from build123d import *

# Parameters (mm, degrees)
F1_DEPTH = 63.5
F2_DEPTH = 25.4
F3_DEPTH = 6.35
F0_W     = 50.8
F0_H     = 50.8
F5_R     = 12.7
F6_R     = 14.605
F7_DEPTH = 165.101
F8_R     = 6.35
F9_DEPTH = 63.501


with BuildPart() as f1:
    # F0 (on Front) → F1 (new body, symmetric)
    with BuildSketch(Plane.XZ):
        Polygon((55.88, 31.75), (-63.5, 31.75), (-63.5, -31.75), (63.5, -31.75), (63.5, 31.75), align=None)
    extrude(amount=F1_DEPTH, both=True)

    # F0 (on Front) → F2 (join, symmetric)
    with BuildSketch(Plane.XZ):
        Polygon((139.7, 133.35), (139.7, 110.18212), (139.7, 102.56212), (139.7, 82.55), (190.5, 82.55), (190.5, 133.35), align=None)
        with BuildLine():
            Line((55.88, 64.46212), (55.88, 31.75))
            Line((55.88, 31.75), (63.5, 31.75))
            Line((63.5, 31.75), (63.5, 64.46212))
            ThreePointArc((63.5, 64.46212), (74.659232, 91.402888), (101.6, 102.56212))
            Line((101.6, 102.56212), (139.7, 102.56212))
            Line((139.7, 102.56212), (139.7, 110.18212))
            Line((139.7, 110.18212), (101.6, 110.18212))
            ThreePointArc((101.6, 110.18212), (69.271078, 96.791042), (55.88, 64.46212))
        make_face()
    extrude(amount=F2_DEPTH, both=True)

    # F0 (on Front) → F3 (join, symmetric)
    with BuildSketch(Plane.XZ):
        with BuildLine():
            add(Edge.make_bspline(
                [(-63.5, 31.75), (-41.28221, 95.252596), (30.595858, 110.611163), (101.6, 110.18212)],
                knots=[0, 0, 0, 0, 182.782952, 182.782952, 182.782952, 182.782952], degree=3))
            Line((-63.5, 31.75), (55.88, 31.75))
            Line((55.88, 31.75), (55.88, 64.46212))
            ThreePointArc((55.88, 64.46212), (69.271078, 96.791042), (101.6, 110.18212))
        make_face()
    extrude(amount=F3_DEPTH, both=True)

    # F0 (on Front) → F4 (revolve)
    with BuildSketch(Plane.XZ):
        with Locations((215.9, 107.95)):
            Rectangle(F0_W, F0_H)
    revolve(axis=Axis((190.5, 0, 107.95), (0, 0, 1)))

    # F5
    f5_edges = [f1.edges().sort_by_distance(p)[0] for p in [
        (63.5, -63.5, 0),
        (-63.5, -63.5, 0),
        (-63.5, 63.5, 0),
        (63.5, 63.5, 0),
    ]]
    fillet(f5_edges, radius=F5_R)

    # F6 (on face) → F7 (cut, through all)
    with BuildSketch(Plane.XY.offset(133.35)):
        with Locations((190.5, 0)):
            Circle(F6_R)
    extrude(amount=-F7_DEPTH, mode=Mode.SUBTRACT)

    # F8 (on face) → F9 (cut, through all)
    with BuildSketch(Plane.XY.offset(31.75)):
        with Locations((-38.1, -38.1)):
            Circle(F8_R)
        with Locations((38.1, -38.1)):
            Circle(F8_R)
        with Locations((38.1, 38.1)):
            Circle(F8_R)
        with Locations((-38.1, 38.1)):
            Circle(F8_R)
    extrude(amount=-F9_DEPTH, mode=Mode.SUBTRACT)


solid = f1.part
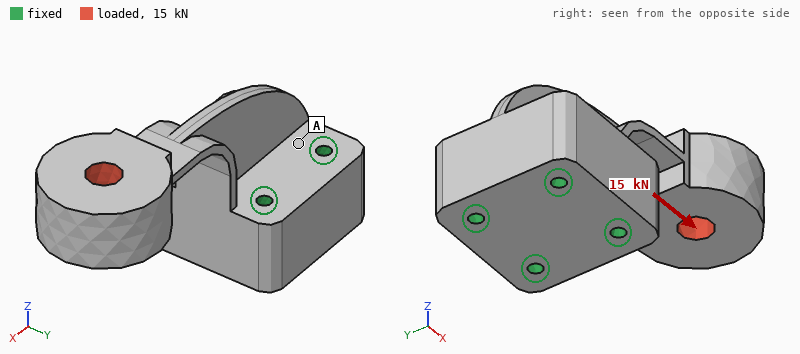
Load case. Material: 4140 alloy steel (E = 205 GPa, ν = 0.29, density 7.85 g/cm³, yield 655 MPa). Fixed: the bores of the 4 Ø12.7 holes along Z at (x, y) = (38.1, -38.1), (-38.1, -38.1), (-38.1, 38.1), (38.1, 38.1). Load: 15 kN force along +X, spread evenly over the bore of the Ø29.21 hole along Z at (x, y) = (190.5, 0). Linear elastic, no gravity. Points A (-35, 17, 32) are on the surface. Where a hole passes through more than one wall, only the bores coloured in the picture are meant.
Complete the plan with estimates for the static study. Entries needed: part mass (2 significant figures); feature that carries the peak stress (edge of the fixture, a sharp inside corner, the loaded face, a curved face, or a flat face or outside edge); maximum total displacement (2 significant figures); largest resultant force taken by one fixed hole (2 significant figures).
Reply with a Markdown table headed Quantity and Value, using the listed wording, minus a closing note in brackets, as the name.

| Quantity | Value |
|---|---|
| part mass | 12 kg |
| feature that carries the peak stress | a curved face |
| maximum total displacement | 0.97 mm |
| largest resultant force taken by one fixed hole | 8.7 kN |
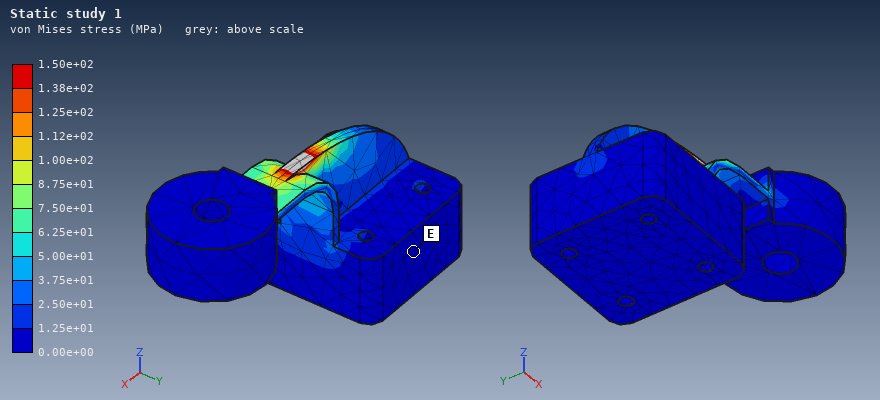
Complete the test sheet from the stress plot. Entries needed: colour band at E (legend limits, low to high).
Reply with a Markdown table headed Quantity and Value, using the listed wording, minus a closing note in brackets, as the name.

| Quantity | Value |
|---|---|
| colour band at E | 0.00e+00 to 1.25e+01 MPa |
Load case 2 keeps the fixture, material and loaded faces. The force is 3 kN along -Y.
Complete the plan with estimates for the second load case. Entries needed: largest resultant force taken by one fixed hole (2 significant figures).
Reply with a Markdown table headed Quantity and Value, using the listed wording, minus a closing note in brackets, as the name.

| Quantity | Value |
|---|---|
| largest resultant force taken by one fixed hole | 6.9 kN |
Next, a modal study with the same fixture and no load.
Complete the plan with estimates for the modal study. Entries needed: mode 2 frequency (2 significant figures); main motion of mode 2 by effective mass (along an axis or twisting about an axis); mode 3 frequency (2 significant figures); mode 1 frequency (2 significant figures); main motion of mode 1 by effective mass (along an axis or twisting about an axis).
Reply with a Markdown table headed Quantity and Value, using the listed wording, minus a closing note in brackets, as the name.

| Quantity | Value |
|---|---|
| mode 2 frequency | 130 Hz |
| main motion of mode 2 by effective mass | along Y |
| mode 3 frequency | 330 Hz |
| mode 1 frequency | 84 Hz |
| main motion of mode 1 by effective mass | along Z |
